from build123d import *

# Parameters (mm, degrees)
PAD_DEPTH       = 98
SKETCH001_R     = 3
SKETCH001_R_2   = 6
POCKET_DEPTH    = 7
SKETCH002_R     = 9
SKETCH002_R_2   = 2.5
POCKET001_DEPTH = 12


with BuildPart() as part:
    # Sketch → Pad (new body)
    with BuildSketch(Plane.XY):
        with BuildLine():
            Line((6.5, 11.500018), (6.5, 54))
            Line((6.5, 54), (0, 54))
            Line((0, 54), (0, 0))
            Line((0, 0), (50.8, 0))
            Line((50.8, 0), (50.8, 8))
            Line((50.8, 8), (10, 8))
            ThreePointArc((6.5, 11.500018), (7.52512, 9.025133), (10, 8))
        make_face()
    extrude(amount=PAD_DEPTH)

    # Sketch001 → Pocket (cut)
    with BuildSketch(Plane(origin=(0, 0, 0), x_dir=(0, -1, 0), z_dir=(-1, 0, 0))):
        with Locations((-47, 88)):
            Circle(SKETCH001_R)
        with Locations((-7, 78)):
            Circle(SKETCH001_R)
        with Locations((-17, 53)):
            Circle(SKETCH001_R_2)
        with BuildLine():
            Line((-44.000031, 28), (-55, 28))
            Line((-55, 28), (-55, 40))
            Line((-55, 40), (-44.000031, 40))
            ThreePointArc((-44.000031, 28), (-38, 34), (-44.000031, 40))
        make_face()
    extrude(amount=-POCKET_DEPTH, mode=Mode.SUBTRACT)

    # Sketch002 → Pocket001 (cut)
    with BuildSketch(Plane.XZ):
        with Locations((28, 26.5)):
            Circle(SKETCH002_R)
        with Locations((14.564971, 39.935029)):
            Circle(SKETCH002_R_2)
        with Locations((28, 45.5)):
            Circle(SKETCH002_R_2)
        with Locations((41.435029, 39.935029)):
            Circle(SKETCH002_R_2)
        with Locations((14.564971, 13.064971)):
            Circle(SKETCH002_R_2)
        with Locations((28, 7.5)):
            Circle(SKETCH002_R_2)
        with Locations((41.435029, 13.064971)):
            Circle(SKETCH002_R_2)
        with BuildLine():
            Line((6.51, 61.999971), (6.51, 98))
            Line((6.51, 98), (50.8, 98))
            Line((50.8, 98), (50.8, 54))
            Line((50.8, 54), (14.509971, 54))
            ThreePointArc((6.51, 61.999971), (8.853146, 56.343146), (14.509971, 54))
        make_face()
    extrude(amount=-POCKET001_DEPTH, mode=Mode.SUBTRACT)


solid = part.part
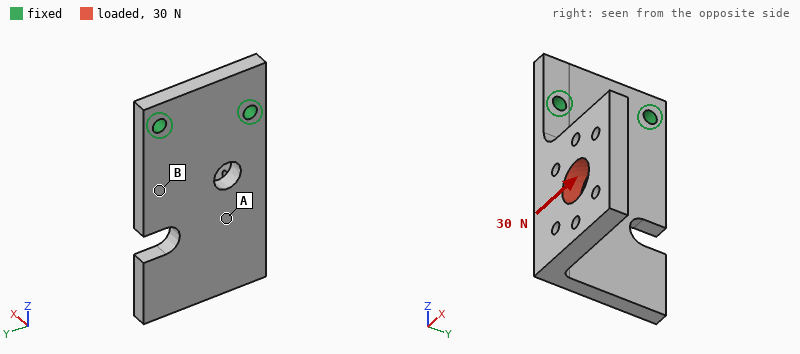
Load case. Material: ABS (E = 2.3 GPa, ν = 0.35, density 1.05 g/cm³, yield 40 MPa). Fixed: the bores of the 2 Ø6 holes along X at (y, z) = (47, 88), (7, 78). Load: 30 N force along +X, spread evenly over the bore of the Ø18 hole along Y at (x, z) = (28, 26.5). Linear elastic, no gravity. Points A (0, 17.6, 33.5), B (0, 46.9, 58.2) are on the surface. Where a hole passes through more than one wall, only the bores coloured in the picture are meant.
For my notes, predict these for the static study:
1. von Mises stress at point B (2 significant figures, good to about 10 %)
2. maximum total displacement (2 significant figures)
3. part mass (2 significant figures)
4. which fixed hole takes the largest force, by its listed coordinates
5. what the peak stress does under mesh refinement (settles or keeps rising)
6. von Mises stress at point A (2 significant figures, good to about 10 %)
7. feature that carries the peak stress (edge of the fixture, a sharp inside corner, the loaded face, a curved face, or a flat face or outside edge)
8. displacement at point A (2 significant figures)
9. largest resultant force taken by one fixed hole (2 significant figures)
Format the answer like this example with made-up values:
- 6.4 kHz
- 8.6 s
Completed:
- 1.9 MPa
- 1.4 mm
- 51 g
- (7, 78)
- keeps rising
- 0.77 MPa
- edge of the fixture
- 0.50 mm
- 39 N
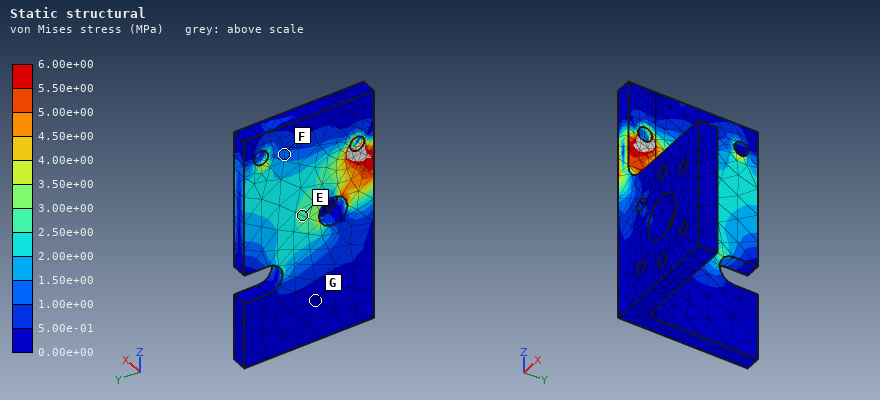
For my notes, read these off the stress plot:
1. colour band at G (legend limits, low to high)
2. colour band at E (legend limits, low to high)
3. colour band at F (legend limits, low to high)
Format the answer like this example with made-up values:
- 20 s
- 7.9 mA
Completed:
- 0.00e+00 to 5.00e-01 MPa
- 2.50e+00 to 3.00e+00 MPa
- 1.00e+00 to 1.50e+00 MPa
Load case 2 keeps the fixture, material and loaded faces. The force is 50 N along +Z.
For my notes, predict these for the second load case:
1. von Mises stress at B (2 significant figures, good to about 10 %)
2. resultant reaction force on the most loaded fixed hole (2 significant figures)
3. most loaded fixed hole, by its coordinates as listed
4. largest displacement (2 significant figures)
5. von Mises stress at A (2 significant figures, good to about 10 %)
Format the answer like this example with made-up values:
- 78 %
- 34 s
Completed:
- 2.1 MPa
- 53 N
- (7, 78)
- 1.4 mm
- 0.91 MPa
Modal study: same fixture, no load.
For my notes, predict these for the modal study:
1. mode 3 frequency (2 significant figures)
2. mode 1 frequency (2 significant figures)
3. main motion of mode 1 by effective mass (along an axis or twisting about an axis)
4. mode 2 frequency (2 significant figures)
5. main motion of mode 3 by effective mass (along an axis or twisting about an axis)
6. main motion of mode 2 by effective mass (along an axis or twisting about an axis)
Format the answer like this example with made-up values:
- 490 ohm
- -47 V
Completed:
- 880 Hz
- 160 Hz
- along X
- 320 Hz
- along Y
- along Y
